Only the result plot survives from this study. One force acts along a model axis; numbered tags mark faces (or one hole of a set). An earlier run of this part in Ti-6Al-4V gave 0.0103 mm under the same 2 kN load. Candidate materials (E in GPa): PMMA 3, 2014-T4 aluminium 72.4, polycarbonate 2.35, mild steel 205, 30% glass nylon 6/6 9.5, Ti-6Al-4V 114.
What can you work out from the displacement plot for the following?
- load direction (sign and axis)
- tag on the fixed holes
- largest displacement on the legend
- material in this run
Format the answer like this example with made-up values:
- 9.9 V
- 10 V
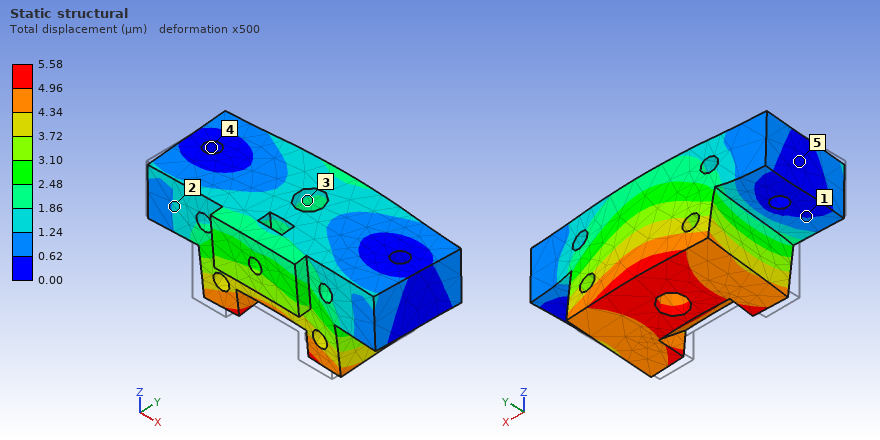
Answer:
- +Y
- 4
- 5.58 µm
- mild steel
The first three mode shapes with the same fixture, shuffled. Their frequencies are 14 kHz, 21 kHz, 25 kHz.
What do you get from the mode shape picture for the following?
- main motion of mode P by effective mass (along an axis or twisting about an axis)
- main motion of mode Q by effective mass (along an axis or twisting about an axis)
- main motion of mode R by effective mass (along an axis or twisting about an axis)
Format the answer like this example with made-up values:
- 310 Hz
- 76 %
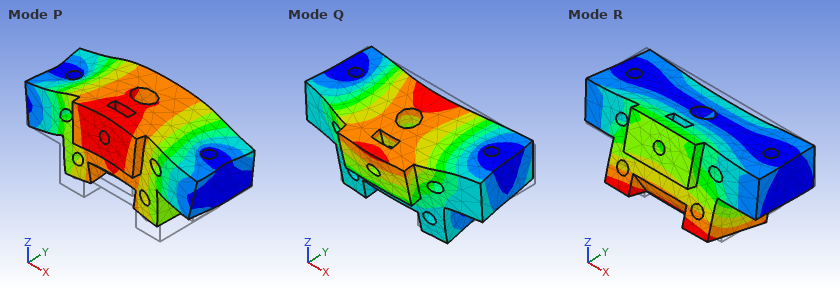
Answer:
- along Z
- along Y
- along Y
